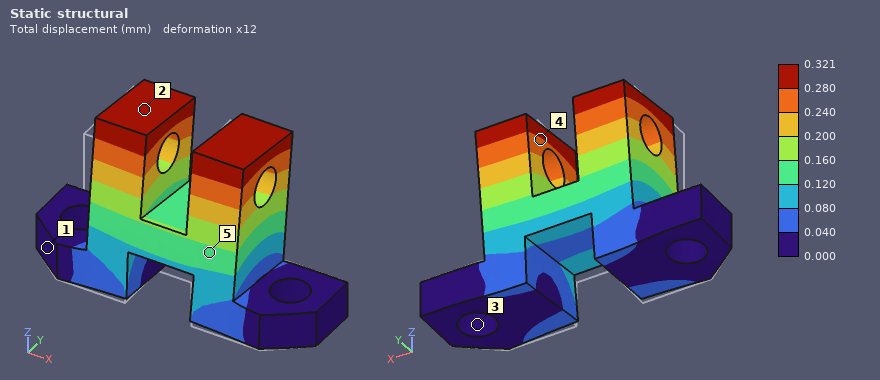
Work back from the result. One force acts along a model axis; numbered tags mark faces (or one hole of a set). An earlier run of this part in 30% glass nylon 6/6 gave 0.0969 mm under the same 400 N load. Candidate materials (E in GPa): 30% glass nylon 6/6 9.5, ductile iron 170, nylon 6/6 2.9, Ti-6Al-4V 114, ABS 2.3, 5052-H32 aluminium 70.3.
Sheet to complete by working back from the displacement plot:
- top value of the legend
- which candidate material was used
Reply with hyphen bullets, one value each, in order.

- 0.321 mm
- nylon 6/6
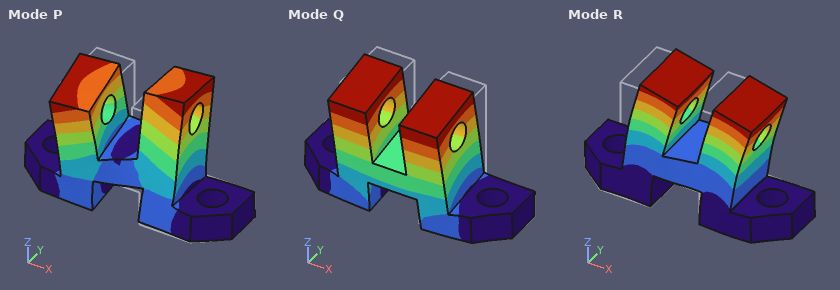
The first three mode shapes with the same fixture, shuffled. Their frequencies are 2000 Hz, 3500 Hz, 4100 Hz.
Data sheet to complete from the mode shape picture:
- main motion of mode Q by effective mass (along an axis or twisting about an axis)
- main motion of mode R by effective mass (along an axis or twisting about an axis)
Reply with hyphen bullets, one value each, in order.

- along Y
- along X
